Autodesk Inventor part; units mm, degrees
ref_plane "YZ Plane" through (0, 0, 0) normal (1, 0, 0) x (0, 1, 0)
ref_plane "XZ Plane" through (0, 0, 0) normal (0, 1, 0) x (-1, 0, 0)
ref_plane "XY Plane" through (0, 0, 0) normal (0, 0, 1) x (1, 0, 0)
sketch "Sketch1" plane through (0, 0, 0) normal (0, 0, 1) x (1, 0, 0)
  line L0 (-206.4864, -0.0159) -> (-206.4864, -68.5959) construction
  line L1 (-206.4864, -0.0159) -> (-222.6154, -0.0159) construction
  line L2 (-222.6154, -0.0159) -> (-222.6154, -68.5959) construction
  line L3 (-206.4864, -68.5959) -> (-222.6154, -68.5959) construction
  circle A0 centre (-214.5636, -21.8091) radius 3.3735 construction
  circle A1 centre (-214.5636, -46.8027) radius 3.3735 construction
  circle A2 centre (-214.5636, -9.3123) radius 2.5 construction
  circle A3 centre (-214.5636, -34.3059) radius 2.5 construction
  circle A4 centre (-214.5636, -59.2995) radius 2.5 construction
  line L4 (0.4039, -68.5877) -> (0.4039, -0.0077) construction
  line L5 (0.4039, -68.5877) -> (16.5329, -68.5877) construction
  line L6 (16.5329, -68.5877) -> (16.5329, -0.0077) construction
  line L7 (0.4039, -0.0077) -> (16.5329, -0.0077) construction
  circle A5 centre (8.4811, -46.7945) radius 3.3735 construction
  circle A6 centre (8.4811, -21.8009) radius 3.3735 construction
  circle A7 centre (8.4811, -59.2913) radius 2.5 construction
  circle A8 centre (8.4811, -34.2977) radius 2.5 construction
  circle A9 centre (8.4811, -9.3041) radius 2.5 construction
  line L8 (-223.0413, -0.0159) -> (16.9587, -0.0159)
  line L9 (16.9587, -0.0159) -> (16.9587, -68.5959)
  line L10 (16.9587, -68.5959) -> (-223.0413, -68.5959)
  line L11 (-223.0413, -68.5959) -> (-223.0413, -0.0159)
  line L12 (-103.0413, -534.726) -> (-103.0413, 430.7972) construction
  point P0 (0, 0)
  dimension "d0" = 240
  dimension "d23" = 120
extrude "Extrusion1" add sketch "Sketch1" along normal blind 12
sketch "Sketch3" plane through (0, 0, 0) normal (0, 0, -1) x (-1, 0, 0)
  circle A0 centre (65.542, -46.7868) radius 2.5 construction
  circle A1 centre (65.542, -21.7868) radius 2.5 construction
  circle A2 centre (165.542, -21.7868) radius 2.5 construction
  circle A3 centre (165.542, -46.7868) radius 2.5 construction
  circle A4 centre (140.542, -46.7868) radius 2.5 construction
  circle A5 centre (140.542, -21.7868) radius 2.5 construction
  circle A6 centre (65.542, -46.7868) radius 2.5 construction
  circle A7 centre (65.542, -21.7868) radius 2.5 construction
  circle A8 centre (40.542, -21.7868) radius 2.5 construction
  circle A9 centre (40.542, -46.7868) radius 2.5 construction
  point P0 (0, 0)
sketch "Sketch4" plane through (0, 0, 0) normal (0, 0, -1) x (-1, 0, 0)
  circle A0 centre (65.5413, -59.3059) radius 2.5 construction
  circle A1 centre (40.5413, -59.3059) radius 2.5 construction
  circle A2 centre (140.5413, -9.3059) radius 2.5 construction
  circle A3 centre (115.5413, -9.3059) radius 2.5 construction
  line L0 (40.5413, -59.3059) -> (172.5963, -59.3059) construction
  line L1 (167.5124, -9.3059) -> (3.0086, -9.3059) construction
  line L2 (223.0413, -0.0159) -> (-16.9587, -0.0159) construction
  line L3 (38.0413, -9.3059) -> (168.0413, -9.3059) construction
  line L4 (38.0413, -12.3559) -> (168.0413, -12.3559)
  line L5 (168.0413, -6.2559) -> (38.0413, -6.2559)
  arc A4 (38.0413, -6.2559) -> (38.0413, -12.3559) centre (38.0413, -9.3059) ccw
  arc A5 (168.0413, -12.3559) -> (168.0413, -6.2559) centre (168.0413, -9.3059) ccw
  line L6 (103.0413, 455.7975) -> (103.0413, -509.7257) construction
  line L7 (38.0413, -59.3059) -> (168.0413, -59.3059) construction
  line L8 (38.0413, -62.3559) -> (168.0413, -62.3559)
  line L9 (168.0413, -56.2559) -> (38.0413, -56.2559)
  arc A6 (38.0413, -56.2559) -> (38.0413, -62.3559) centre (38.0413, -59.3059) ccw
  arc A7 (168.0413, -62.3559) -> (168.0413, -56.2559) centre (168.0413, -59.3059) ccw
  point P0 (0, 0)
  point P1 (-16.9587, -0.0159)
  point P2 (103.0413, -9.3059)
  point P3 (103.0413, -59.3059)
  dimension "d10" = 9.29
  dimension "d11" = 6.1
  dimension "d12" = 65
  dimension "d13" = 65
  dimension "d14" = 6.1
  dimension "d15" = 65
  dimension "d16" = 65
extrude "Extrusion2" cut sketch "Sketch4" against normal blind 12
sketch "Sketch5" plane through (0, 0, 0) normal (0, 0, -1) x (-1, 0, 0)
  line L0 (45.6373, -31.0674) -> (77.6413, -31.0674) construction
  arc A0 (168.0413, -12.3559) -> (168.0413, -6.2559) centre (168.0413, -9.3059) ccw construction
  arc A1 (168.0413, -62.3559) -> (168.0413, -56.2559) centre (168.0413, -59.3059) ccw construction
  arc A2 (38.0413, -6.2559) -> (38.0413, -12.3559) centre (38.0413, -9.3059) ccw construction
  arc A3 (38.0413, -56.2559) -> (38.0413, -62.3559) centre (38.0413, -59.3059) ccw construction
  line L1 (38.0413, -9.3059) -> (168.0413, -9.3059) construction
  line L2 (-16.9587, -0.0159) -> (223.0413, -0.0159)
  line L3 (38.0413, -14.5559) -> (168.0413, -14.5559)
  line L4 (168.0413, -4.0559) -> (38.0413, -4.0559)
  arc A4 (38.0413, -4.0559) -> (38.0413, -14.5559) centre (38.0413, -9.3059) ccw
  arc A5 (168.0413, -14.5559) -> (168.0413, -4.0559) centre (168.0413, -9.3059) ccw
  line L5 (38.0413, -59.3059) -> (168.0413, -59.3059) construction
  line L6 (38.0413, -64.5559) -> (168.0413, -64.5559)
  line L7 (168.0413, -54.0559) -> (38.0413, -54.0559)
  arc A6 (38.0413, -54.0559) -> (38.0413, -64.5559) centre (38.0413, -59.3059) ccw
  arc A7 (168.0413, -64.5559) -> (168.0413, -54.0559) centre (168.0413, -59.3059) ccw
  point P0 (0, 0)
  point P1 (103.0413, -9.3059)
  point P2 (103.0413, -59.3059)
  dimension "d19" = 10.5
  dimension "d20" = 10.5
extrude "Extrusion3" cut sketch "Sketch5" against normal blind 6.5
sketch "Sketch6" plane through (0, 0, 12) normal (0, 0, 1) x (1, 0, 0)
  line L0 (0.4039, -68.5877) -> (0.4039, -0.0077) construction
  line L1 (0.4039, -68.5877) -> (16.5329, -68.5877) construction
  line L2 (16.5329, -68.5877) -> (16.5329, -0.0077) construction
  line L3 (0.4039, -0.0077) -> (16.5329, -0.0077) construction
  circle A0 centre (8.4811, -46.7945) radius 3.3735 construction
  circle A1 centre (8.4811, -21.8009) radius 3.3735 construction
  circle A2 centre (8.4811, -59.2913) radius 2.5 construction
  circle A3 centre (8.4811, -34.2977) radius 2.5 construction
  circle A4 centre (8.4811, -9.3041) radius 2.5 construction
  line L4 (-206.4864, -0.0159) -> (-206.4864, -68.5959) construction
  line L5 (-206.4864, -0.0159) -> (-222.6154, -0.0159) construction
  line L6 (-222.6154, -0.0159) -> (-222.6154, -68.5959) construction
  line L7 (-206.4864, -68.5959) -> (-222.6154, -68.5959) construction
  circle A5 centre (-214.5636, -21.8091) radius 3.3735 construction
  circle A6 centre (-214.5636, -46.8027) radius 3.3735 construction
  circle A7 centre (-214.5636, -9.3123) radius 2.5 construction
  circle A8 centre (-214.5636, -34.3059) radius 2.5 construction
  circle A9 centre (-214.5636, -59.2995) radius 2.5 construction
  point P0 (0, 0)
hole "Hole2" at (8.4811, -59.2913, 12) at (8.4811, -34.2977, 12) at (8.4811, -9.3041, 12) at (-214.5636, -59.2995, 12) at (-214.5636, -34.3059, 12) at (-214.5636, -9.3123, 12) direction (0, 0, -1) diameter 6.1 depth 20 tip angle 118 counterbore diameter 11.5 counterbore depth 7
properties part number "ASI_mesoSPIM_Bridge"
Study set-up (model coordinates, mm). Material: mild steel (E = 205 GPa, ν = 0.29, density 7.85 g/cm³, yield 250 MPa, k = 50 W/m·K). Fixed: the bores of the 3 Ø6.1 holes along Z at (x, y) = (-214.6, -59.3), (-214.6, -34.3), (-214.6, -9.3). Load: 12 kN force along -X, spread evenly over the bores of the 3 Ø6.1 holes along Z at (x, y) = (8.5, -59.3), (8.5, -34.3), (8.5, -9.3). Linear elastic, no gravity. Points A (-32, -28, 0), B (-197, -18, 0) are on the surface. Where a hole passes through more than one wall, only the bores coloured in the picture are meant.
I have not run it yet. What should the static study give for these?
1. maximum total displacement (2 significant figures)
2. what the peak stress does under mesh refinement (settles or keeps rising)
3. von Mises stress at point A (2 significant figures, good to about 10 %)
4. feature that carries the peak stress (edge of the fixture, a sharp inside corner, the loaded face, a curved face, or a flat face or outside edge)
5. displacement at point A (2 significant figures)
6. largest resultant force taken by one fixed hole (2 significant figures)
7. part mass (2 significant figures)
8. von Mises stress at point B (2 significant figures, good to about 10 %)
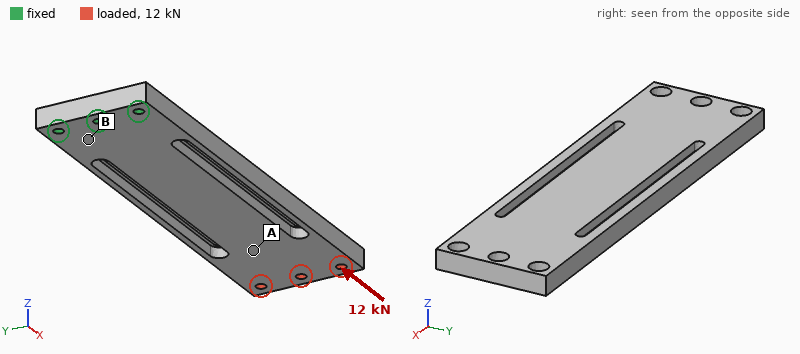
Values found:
0.69 mm
keeps rising
50 MPa
edge of the fixture
0.42 mm
4.3 kN
1.3 kg
38 MPa
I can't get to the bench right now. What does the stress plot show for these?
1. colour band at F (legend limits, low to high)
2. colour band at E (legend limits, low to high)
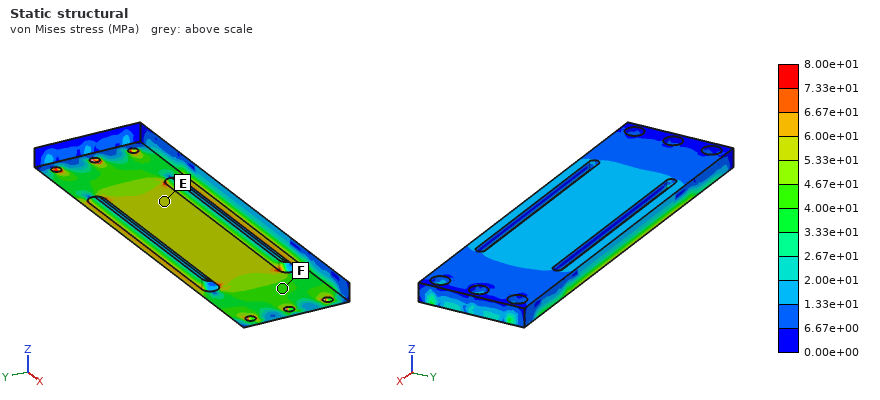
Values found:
4.00e+01 to 4.67e+01 MPa
5.33e+01 to 6.00e+01 MPa
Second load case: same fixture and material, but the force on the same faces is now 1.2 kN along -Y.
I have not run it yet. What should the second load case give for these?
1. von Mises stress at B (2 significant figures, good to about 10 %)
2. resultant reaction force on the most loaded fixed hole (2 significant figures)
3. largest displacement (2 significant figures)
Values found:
27 MPa
5.1 kN
0.15 mm
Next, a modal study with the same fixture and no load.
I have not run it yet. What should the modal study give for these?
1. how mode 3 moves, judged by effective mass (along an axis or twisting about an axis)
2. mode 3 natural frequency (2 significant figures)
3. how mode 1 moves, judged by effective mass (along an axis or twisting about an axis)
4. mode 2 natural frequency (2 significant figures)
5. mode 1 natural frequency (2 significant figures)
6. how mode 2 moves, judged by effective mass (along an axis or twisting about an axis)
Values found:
along Z
1000 Hz
along Z
760 Hz
160 Hz
along Y
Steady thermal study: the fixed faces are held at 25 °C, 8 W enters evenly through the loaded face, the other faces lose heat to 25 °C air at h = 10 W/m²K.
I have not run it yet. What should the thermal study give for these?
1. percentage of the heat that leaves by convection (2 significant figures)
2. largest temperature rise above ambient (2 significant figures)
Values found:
66 %
30 K
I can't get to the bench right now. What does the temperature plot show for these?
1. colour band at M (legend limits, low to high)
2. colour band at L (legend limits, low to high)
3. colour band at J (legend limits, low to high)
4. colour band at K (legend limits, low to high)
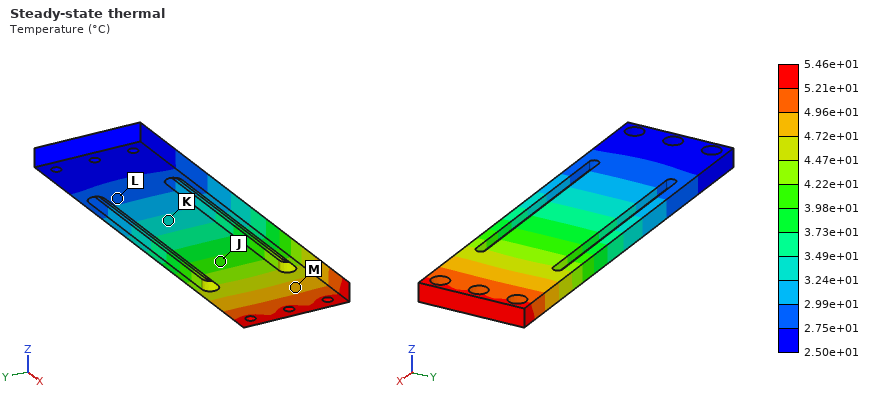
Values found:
4.72e+01 to 4.96e+01 °C
2.75e+01 to 2.99e+01 °C
3.98e+01 to 4.22e+01 °C
3.24e+01 to 3.49e+01 °C
